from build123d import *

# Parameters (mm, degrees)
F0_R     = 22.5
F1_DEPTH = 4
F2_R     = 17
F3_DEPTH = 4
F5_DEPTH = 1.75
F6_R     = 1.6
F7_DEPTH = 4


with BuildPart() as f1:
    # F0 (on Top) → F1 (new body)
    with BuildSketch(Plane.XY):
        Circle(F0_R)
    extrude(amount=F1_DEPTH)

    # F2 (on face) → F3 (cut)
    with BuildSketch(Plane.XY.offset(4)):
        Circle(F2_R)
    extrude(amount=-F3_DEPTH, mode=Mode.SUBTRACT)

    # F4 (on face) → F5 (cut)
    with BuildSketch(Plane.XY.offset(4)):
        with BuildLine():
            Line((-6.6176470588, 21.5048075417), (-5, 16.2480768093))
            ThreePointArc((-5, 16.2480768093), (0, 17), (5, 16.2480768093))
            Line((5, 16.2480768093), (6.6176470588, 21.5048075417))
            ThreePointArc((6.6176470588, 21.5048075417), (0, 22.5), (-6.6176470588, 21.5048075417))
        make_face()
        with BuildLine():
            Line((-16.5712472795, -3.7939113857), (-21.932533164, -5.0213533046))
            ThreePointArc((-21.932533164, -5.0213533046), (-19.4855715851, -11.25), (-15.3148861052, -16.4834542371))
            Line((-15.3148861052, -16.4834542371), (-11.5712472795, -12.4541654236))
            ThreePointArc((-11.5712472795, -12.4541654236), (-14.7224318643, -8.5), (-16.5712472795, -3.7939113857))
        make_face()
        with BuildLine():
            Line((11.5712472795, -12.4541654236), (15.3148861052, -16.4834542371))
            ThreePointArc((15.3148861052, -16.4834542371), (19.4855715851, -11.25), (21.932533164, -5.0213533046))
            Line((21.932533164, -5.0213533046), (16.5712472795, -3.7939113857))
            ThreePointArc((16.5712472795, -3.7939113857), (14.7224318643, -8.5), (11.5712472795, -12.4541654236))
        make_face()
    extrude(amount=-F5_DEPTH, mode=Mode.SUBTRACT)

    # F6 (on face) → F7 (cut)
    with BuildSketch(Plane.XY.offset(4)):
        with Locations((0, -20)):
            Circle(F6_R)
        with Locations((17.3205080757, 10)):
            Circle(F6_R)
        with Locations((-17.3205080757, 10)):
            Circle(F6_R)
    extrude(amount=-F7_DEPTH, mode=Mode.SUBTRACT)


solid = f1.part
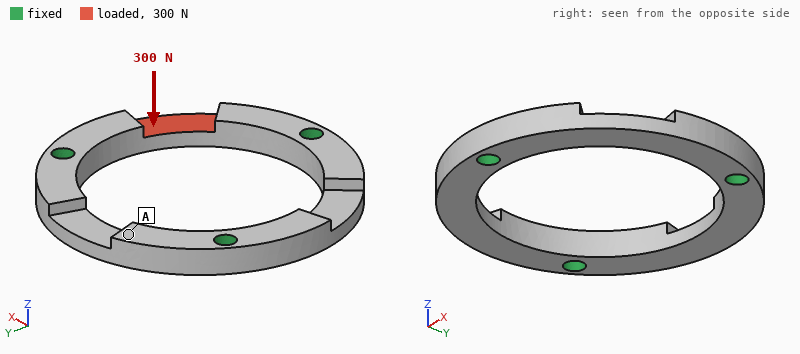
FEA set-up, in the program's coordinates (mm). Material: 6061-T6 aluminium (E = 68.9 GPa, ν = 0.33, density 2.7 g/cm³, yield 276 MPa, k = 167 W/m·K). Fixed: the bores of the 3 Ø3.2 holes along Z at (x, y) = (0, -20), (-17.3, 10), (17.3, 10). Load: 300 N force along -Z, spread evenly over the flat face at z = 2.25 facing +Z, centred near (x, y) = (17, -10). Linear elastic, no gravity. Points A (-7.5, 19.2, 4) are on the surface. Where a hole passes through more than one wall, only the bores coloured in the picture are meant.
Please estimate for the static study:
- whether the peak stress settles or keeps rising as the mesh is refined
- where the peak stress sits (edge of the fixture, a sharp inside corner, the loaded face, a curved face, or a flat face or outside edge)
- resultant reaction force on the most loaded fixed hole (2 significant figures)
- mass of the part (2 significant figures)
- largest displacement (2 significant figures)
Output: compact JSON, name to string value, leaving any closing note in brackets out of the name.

{"whether the peak stress settles or keeps rising as the mesh is refined": "keeps rising", "where the peak stress sits": "edge of the fixture", "resultant reaction force on the most loaded fixed hole": "160 N", "mass of the part": "6.2 g", "largest displacement": "0.11 mm"}
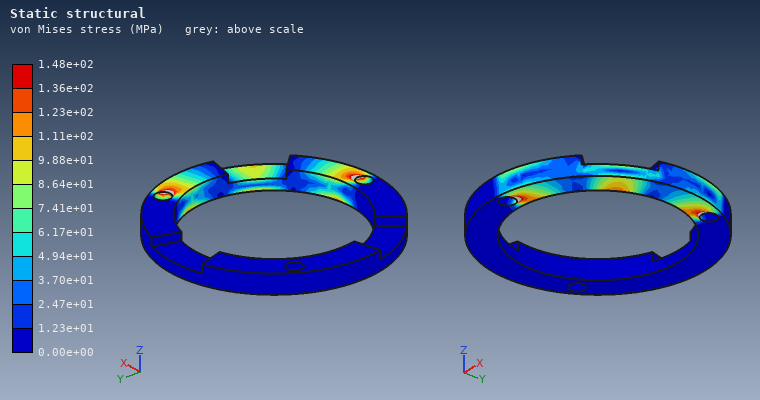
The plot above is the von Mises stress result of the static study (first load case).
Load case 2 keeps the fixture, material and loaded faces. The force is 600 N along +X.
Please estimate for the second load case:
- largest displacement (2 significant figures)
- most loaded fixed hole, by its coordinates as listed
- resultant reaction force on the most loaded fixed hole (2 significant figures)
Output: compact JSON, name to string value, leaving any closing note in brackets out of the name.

{"largest displacement": "27 µm", "most loaded fixed hole, by its coordinates as listed": "(0, -20)", "resultant reaction force on the most loaded fixed hole": "560 N"}
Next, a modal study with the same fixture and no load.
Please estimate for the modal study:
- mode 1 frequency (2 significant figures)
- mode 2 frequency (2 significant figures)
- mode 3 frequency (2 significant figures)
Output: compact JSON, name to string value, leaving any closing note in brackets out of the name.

{"mode 1 frequency": "12 kHz", "mode 2 frequency": "12 kHz", "mode 3 frequency": "12 kHz"}
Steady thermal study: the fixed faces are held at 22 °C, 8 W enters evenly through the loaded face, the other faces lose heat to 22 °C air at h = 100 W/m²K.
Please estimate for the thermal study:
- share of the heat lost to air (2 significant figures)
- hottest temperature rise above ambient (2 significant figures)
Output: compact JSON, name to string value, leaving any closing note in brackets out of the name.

{"share of the heat lost to air": "7.5 %", "hottest temperature rise above ambient": "21 K"}
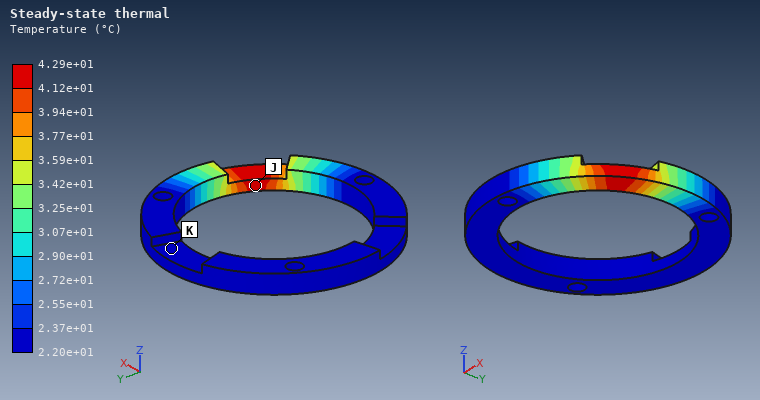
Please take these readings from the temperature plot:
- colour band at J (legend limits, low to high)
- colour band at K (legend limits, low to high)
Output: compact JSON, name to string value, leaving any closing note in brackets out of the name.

{"colour band at J": "4.12e+01 to 4.29e+01 °C", "colour band at K": "2.20e+01 to 2.37e+01 °C"}
